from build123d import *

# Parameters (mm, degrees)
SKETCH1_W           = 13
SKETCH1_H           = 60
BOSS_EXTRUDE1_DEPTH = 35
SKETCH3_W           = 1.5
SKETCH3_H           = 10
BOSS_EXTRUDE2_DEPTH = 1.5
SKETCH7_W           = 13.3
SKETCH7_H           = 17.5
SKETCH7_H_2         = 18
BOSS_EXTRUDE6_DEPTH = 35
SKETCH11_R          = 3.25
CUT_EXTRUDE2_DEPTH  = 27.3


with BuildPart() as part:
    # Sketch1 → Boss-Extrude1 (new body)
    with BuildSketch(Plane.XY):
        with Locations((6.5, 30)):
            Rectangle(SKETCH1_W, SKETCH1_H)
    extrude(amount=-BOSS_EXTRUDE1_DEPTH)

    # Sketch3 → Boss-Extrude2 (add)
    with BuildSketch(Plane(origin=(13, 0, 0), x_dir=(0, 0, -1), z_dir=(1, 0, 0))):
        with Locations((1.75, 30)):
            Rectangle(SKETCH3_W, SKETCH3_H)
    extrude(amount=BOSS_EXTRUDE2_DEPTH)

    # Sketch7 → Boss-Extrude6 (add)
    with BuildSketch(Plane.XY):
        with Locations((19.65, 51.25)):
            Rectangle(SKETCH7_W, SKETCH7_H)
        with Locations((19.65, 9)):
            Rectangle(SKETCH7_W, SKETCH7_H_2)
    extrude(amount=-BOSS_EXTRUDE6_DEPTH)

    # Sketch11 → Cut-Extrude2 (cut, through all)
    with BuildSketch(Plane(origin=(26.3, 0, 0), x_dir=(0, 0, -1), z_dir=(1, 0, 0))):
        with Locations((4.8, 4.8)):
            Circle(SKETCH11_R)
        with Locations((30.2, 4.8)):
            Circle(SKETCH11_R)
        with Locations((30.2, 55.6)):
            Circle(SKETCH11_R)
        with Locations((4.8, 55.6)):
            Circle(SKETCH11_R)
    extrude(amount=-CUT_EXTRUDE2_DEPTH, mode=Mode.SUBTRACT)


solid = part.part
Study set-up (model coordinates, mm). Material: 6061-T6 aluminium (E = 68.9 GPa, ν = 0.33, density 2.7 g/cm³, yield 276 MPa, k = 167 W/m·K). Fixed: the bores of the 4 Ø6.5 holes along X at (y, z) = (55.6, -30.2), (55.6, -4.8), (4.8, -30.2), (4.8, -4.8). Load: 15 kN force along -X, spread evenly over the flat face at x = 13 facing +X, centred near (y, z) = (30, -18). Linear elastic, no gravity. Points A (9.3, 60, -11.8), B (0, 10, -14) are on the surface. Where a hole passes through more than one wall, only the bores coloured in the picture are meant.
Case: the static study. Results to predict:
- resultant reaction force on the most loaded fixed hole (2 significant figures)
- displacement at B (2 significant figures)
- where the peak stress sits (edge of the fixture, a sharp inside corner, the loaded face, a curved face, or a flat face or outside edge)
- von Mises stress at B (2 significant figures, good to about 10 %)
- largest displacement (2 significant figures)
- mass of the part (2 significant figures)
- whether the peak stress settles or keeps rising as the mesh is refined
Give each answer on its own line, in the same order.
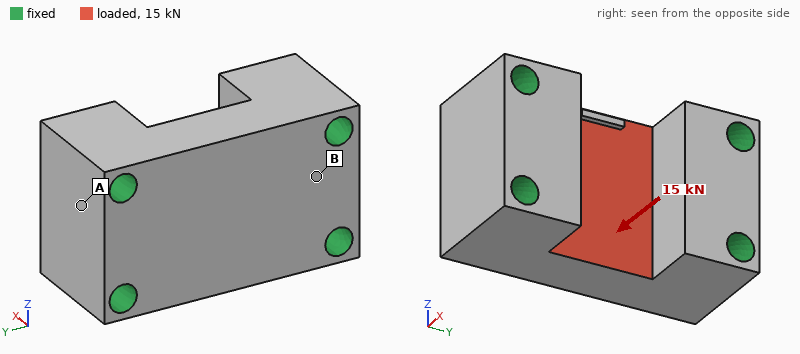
3.9 kN
4.5 µm
edge of the fixture
12 MPa
19 µm
110 g
keeps rising
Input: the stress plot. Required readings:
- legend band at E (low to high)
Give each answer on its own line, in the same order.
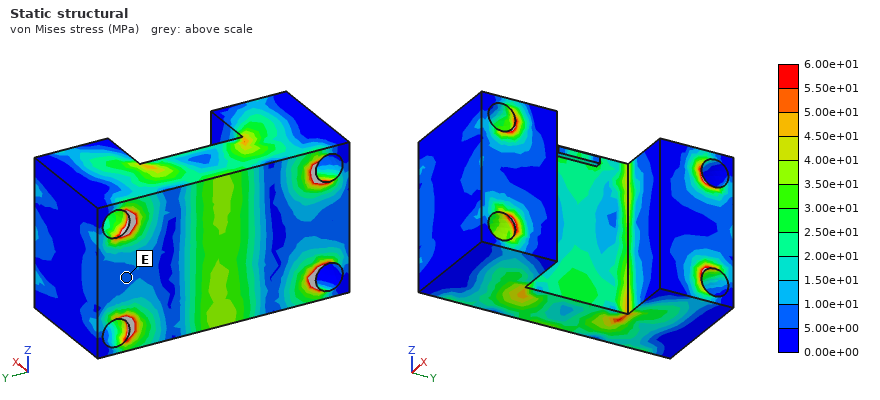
5.00e+00 to 1.00e+01 MPa
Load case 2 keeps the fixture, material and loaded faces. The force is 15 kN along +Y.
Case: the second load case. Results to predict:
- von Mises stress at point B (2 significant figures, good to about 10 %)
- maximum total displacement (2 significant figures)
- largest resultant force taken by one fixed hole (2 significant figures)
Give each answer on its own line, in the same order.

5.9 MPa
8.1 µm
4.0 kN
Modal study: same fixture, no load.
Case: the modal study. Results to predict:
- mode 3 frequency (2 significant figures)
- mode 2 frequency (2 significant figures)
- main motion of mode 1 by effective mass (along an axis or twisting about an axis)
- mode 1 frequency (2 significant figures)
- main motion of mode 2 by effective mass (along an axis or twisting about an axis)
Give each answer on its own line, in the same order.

35 kHz
31 kHz
along X
28 kHz
along Z
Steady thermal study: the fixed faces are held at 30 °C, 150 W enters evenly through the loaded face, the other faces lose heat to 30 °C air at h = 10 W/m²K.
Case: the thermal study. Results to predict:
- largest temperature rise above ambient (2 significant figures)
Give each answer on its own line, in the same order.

19 K
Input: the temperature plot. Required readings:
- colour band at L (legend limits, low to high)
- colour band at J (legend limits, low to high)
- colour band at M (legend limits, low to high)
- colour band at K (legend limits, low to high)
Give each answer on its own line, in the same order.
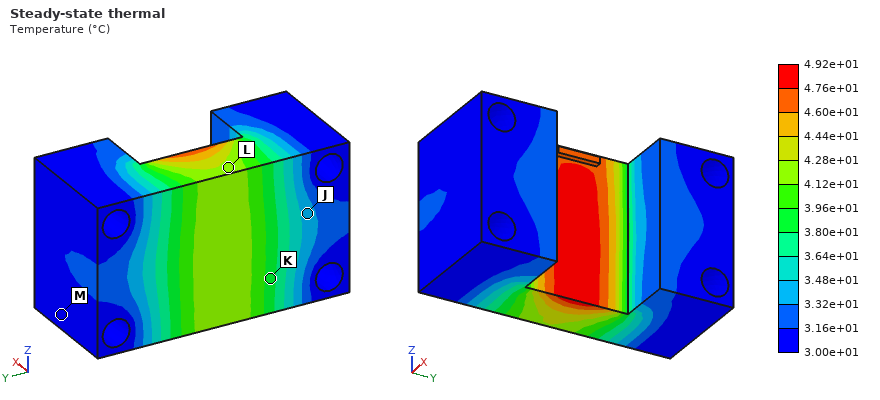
4.12e+01 to 4.28e+01 °C
3.32e+01 to 3.48e+01 °C
3.00e+01 to 3.16e+01 °C
3.80e+01 to 3.96e+01 °C
